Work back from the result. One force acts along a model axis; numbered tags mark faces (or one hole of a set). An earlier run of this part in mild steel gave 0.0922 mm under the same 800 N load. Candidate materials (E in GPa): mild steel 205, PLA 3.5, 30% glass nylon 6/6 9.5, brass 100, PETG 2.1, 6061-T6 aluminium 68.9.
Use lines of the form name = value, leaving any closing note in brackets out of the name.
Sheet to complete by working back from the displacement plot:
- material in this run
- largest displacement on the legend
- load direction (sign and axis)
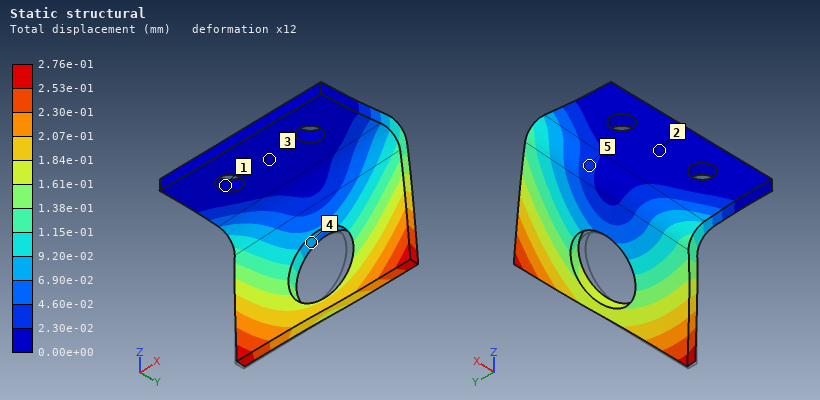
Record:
material in this run = 6061-T6 aluminium
largest displacement on the legend = 2.76e-01 mm
load direction = +X
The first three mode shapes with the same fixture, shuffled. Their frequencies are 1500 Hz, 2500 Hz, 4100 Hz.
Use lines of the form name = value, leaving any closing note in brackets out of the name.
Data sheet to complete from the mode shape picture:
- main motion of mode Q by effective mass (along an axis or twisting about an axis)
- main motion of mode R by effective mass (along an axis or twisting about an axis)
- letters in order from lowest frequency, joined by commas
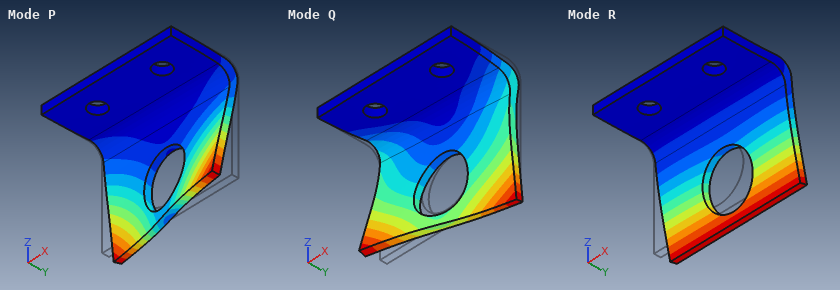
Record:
main motion of mode Q by effective mass = along X
main motion of mode R by effective mass = along Y
letters in order from lowest frequency, joined by commas = R, P, Q
